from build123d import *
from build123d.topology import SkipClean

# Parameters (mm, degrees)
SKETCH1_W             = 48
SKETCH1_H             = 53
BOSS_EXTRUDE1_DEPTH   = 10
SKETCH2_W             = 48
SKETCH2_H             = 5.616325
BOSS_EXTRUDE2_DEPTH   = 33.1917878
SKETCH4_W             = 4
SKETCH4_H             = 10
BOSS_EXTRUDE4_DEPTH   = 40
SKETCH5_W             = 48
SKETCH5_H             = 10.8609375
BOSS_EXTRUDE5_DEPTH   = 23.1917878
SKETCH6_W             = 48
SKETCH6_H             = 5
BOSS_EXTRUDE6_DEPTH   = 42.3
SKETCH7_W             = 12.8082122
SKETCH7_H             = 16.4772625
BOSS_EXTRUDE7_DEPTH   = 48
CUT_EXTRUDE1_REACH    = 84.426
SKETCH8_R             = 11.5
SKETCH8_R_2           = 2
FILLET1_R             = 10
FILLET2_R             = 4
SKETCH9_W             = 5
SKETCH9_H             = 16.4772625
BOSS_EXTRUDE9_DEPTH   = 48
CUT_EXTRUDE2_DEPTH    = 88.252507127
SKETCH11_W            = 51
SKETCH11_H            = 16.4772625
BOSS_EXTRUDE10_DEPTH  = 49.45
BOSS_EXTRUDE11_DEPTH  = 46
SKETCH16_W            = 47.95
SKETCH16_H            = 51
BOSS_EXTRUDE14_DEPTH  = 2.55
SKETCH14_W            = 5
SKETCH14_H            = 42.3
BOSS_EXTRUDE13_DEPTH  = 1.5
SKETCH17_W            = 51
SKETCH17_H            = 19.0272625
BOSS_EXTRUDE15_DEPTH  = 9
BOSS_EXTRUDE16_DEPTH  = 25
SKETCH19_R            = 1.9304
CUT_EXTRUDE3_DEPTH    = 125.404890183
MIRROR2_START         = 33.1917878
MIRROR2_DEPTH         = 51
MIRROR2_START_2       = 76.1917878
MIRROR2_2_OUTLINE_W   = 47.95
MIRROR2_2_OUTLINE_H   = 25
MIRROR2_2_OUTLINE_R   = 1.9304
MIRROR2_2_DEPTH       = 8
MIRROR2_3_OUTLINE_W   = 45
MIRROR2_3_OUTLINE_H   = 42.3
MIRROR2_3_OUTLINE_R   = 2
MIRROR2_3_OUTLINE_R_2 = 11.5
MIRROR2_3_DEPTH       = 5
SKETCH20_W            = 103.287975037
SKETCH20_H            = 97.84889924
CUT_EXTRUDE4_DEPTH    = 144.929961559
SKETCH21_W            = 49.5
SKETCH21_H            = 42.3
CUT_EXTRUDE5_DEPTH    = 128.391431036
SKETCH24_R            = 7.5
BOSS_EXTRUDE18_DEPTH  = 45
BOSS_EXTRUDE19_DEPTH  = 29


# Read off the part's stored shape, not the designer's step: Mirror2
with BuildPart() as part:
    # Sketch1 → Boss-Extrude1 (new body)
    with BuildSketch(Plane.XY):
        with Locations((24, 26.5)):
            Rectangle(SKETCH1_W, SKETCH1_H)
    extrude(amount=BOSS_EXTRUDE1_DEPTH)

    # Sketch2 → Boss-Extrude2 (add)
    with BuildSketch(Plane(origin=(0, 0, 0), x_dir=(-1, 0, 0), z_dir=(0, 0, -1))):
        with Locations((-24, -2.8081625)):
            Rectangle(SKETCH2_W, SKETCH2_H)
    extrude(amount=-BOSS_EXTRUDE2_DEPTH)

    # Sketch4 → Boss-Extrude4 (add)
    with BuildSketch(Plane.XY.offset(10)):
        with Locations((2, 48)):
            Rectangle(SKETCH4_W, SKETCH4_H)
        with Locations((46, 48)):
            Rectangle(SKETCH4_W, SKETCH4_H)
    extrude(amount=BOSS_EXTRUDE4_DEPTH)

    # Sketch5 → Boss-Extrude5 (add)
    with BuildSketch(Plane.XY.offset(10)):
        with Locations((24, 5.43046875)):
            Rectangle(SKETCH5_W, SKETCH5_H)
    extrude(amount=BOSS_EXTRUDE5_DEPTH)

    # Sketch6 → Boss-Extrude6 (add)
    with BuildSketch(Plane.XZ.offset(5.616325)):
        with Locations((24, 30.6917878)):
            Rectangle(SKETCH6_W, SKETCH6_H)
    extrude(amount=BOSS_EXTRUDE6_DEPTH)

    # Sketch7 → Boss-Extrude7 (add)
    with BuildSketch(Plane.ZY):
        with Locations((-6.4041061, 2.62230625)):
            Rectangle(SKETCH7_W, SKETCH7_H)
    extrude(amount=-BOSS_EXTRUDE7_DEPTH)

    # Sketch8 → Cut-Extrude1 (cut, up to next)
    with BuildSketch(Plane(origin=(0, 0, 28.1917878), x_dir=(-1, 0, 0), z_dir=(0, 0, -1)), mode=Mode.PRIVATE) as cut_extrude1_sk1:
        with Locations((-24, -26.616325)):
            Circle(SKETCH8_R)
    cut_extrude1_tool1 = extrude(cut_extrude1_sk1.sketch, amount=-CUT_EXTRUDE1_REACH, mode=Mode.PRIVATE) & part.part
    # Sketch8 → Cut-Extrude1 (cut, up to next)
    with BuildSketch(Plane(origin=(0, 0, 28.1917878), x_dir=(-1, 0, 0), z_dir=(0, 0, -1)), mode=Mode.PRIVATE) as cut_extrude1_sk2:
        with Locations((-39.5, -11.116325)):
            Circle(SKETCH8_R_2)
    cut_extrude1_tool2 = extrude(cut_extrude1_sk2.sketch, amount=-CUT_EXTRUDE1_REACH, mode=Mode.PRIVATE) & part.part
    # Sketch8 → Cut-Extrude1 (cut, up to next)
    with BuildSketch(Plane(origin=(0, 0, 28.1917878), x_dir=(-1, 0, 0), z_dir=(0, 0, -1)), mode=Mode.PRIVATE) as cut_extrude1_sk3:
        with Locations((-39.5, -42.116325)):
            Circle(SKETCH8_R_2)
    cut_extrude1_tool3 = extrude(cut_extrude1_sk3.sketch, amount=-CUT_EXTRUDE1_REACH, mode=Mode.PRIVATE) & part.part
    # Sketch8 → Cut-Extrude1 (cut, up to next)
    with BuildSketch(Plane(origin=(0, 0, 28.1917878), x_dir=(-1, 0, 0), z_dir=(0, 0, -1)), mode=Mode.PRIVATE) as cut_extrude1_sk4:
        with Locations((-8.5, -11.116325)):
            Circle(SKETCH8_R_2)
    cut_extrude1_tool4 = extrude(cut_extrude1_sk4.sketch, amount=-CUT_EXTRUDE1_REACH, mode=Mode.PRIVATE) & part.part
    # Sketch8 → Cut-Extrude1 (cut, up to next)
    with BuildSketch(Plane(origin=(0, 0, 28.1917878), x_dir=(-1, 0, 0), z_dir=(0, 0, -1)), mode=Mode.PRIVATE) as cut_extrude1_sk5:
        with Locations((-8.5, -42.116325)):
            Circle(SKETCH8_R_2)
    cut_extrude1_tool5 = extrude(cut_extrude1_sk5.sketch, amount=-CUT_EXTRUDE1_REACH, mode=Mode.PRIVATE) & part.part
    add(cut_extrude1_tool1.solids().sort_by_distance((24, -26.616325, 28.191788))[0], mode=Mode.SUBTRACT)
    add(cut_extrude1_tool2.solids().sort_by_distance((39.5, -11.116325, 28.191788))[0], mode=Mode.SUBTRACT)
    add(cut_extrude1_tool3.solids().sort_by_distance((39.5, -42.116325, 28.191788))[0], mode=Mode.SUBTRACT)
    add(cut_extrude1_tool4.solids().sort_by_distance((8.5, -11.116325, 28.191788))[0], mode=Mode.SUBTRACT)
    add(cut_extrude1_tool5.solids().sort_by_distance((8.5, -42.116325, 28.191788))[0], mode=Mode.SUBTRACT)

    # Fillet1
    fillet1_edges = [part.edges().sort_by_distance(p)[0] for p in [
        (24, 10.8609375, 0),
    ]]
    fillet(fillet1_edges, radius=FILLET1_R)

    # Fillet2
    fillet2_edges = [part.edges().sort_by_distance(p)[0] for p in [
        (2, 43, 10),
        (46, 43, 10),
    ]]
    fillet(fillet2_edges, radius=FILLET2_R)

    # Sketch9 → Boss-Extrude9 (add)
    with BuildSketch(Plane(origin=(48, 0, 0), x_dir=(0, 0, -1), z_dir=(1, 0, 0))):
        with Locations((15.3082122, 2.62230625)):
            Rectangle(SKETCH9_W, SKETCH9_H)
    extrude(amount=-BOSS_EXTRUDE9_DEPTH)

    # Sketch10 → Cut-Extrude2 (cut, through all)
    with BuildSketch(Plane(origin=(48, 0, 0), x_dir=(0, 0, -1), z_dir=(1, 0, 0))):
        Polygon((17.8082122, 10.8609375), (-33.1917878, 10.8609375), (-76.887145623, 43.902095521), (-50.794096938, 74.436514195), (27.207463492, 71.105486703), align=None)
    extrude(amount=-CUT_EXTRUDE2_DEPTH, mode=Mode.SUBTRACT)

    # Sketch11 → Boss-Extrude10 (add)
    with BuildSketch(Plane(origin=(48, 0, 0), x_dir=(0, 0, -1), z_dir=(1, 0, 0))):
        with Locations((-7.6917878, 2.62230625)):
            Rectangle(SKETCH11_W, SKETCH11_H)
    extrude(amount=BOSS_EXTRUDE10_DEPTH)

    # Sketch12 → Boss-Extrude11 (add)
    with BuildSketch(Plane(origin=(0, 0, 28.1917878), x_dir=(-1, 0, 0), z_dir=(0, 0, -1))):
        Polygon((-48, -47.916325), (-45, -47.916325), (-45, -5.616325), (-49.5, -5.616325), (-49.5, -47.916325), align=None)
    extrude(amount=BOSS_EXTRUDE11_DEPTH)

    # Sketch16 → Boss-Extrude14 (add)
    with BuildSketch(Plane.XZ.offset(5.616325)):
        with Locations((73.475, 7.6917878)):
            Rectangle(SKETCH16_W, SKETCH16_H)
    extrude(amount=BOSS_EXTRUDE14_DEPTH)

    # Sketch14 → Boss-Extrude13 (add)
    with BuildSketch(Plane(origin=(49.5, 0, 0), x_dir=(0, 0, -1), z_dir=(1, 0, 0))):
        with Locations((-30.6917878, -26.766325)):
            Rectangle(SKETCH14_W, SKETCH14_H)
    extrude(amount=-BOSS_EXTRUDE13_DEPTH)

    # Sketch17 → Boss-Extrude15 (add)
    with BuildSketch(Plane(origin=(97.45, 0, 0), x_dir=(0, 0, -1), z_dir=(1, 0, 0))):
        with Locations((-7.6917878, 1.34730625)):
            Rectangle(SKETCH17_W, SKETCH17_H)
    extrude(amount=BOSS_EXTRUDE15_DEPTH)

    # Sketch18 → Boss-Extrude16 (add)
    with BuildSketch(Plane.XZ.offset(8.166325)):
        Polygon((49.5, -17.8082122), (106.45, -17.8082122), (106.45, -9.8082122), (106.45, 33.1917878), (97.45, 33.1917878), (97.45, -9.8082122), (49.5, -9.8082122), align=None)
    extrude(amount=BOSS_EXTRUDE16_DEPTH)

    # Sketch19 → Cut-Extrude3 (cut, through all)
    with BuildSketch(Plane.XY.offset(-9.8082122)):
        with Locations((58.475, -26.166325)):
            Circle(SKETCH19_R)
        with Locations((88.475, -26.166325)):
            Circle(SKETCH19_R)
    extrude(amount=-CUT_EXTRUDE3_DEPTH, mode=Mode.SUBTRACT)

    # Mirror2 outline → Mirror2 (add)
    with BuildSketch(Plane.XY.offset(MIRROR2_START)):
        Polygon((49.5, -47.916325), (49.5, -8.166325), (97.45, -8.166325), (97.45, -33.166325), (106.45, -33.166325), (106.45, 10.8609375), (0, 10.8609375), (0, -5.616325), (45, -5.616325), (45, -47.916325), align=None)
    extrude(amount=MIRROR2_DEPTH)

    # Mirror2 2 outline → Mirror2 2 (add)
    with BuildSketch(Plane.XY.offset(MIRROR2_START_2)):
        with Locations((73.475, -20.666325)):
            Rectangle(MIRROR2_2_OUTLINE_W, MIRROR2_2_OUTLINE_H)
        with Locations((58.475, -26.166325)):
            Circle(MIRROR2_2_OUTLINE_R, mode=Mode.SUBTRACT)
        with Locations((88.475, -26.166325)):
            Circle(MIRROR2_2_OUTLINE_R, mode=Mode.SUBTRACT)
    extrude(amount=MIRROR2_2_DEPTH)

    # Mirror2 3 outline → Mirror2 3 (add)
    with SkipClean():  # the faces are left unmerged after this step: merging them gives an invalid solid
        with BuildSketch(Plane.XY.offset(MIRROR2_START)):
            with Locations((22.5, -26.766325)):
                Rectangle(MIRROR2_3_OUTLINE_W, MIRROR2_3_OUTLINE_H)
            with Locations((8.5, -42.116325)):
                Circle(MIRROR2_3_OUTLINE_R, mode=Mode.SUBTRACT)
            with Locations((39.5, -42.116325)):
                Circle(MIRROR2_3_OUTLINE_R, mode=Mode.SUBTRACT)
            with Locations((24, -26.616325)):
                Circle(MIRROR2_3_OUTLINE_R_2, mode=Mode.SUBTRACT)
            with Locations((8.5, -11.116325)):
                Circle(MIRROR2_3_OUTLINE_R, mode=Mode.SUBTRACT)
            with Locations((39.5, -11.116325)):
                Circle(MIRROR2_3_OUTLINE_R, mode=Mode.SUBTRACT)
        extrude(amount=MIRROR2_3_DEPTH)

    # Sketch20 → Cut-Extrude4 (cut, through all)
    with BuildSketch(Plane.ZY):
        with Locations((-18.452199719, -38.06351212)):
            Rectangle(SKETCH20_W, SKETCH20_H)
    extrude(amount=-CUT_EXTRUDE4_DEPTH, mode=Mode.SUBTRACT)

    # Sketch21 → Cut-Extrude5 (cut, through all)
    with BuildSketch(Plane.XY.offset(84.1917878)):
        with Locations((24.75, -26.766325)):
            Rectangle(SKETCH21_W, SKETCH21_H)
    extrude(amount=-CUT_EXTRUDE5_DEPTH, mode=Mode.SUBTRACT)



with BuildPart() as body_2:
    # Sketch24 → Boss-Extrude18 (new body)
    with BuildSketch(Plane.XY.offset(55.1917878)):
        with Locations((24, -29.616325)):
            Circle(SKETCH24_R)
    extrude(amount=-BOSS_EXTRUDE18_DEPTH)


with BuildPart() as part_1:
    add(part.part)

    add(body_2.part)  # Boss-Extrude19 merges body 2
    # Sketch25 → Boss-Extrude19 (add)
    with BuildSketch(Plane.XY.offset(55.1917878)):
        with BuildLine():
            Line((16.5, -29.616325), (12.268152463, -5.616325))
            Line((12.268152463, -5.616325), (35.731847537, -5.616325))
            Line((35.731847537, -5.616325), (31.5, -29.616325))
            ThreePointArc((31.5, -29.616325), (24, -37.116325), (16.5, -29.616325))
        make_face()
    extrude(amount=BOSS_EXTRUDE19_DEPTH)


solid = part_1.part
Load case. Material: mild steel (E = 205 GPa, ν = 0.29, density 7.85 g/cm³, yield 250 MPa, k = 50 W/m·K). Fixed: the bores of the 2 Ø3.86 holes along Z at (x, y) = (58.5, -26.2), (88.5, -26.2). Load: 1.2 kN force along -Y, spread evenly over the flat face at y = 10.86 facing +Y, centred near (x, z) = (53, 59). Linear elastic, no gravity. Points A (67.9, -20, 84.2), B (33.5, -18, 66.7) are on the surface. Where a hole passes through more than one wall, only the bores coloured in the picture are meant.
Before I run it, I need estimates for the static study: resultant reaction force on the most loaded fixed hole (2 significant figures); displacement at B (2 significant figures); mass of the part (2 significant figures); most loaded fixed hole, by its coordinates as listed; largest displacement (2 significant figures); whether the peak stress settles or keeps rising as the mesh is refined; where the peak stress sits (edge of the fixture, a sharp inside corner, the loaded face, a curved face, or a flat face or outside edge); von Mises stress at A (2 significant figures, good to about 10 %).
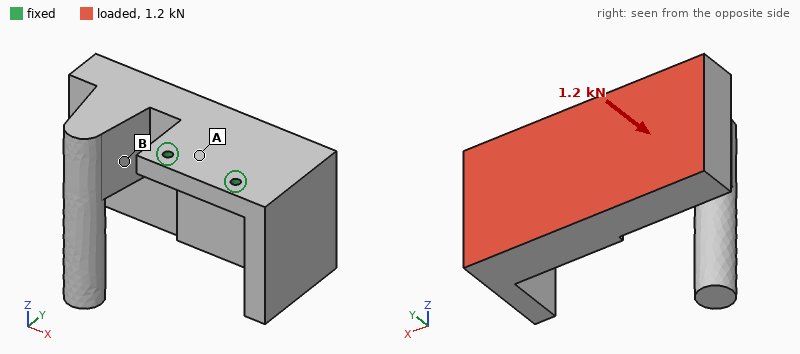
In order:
1.4 kN
18 µm
1.1 kg
(58.5, -26.2)
77 µm
keeps rising
edge of the fixture
22 MPa
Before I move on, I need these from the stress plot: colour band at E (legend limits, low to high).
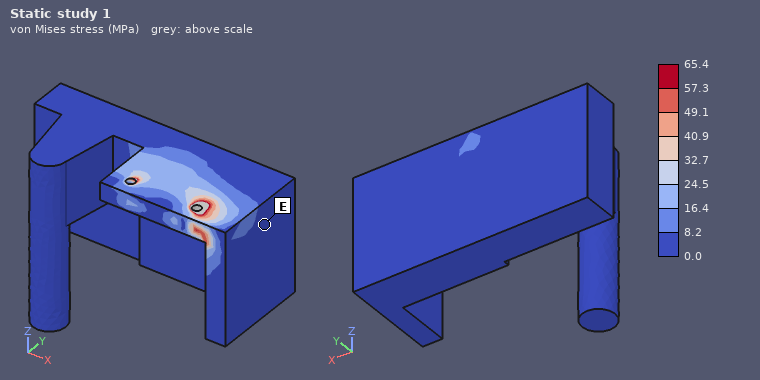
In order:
0.0 to 8.2 MPa
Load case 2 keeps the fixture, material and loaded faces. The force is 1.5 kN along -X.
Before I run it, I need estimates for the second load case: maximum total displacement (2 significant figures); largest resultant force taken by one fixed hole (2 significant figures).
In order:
31 µm
2.1 kN
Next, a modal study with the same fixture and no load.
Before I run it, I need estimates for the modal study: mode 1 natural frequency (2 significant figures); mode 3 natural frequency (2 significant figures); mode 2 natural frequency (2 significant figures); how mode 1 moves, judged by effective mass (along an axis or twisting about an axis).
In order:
790 Hz
1900 Hz
1000 Hz
along Y
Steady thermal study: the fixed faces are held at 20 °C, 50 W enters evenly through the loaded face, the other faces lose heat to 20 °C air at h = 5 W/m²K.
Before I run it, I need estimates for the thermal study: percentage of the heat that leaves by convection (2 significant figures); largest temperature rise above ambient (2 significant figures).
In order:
11 %
74 K
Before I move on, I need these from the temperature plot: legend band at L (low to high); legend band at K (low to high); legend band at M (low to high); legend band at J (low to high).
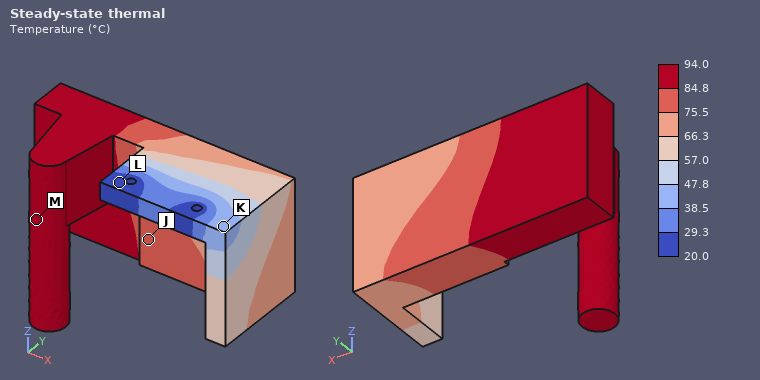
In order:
20.0 to 29.3 °C
38.5 to 47.8 °C
84.8 to 94.0 °C
75.5 to 84.8 °C
